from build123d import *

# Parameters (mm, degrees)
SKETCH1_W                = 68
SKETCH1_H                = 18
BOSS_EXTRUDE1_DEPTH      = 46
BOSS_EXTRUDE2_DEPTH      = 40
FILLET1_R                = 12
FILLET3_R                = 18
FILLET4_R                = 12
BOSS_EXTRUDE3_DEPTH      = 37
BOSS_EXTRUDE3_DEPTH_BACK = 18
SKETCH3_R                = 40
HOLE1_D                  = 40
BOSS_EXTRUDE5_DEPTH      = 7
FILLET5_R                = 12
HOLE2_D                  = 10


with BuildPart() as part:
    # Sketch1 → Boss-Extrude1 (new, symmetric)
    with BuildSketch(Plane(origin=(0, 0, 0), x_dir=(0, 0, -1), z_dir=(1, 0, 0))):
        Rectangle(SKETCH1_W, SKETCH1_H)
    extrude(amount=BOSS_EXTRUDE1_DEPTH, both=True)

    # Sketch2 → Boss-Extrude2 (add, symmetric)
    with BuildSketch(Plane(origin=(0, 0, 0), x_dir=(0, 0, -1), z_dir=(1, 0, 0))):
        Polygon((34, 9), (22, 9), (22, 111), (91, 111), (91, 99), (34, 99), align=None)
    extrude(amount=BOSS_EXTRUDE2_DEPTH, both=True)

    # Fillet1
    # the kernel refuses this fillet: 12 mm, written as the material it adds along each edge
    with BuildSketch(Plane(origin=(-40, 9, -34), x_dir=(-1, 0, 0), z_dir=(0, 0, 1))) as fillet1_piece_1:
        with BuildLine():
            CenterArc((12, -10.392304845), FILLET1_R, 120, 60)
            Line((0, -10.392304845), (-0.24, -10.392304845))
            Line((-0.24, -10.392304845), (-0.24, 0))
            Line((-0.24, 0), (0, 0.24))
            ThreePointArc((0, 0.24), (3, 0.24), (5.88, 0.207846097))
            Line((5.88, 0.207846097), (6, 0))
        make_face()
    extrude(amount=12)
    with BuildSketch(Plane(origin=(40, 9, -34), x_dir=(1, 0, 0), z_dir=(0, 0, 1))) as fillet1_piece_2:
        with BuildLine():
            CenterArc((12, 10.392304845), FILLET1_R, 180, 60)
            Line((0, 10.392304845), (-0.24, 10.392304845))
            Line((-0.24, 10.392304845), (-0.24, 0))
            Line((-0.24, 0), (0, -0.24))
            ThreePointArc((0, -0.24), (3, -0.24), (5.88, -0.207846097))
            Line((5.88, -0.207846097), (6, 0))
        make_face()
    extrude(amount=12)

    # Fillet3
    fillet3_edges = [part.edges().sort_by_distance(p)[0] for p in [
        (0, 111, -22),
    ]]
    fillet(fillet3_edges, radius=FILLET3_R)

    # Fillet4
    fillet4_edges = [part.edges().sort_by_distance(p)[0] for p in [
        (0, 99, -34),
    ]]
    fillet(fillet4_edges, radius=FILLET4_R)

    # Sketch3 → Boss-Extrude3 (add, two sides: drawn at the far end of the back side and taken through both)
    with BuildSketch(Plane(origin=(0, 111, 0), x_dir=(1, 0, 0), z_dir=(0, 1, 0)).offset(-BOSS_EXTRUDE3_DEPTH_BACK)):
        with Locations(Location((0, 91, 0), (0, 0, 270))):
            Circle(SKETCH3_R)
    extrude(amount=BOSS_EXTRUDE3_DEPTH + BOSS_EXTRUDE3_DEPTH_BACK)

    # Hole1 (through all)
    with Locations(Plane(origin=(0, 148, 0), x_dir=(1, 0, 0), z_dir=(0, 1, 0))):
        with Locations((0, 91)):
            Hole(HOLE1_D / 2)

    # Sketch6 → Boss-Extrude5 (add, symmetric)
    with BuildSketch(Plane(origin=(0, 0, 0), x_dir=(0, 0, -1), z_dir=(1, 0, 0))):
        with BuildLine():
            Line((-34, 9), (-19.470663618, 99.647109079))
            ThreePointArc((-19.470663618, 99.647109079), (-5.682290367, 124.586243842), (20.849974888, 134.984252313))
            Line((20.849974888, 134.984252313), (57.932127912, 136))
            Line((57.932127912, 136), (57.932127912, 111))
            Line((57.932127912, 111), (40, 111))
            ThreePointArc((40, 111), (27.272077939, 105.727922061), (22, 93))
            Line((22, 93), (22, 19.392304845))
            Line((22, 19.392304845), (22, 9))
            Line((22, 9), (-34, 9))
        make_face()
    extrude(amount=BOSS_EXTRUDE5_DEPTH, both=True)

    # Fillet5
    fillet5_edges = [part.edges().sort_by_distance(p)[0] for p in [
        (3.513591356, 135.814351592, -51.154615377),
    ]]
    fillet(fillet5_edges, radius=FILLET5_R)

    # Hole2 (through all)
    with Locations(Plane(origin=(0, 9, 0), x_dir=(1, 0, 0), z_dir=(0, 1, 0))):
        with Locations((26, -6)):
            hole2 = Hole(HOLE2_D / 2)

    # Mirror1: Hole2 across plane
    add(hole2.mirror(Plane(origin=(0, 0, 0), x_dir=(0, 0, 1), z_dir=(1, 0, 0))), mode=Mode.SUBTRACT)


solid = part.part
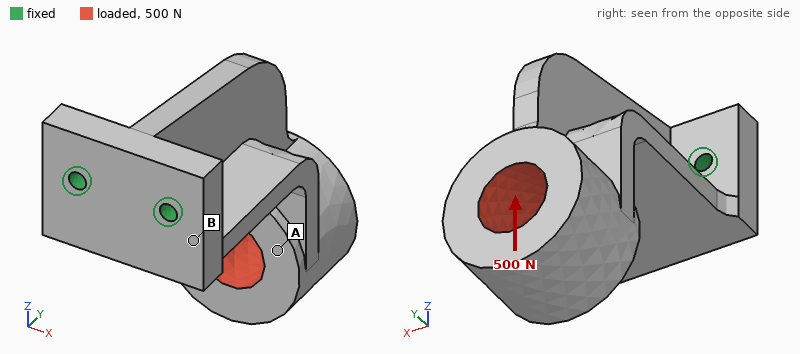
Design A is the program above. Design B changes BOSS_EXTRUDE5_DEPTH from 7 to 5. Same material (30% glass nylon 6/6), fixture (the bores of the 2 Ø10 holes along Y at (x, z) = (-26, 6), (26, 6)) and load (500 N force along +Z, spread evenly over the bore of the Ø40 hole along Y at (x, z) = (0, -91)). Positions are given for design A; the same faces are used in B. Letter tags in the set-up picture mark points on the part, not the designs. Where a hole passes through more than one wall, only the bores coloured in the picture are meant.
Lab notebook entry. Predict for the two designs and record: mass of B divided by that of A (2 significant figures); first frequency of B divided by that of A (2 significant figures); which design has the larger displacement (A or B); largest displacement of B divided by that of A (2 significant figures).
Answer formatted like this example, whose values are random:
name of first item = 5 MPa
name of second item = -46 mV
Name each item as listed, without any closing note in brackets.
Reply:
mass of B divided by that of A = 0.95
first frequency of B divided by that of A = 0.91
which design has the larger displacement = B
largest displacement of B divided by that of A = 1.1
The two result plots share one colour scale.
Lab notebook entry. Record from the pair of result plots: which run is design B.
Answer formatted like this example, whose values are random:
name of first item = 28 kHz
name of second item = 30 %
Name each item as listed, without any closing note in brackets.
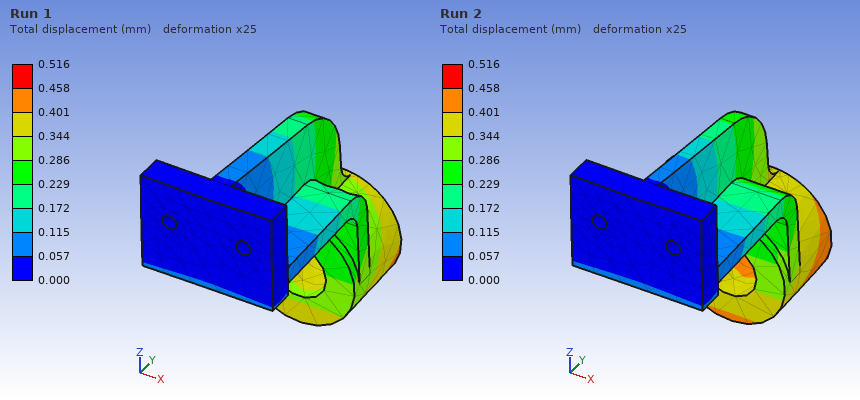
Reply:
which run is design B = Run 2
